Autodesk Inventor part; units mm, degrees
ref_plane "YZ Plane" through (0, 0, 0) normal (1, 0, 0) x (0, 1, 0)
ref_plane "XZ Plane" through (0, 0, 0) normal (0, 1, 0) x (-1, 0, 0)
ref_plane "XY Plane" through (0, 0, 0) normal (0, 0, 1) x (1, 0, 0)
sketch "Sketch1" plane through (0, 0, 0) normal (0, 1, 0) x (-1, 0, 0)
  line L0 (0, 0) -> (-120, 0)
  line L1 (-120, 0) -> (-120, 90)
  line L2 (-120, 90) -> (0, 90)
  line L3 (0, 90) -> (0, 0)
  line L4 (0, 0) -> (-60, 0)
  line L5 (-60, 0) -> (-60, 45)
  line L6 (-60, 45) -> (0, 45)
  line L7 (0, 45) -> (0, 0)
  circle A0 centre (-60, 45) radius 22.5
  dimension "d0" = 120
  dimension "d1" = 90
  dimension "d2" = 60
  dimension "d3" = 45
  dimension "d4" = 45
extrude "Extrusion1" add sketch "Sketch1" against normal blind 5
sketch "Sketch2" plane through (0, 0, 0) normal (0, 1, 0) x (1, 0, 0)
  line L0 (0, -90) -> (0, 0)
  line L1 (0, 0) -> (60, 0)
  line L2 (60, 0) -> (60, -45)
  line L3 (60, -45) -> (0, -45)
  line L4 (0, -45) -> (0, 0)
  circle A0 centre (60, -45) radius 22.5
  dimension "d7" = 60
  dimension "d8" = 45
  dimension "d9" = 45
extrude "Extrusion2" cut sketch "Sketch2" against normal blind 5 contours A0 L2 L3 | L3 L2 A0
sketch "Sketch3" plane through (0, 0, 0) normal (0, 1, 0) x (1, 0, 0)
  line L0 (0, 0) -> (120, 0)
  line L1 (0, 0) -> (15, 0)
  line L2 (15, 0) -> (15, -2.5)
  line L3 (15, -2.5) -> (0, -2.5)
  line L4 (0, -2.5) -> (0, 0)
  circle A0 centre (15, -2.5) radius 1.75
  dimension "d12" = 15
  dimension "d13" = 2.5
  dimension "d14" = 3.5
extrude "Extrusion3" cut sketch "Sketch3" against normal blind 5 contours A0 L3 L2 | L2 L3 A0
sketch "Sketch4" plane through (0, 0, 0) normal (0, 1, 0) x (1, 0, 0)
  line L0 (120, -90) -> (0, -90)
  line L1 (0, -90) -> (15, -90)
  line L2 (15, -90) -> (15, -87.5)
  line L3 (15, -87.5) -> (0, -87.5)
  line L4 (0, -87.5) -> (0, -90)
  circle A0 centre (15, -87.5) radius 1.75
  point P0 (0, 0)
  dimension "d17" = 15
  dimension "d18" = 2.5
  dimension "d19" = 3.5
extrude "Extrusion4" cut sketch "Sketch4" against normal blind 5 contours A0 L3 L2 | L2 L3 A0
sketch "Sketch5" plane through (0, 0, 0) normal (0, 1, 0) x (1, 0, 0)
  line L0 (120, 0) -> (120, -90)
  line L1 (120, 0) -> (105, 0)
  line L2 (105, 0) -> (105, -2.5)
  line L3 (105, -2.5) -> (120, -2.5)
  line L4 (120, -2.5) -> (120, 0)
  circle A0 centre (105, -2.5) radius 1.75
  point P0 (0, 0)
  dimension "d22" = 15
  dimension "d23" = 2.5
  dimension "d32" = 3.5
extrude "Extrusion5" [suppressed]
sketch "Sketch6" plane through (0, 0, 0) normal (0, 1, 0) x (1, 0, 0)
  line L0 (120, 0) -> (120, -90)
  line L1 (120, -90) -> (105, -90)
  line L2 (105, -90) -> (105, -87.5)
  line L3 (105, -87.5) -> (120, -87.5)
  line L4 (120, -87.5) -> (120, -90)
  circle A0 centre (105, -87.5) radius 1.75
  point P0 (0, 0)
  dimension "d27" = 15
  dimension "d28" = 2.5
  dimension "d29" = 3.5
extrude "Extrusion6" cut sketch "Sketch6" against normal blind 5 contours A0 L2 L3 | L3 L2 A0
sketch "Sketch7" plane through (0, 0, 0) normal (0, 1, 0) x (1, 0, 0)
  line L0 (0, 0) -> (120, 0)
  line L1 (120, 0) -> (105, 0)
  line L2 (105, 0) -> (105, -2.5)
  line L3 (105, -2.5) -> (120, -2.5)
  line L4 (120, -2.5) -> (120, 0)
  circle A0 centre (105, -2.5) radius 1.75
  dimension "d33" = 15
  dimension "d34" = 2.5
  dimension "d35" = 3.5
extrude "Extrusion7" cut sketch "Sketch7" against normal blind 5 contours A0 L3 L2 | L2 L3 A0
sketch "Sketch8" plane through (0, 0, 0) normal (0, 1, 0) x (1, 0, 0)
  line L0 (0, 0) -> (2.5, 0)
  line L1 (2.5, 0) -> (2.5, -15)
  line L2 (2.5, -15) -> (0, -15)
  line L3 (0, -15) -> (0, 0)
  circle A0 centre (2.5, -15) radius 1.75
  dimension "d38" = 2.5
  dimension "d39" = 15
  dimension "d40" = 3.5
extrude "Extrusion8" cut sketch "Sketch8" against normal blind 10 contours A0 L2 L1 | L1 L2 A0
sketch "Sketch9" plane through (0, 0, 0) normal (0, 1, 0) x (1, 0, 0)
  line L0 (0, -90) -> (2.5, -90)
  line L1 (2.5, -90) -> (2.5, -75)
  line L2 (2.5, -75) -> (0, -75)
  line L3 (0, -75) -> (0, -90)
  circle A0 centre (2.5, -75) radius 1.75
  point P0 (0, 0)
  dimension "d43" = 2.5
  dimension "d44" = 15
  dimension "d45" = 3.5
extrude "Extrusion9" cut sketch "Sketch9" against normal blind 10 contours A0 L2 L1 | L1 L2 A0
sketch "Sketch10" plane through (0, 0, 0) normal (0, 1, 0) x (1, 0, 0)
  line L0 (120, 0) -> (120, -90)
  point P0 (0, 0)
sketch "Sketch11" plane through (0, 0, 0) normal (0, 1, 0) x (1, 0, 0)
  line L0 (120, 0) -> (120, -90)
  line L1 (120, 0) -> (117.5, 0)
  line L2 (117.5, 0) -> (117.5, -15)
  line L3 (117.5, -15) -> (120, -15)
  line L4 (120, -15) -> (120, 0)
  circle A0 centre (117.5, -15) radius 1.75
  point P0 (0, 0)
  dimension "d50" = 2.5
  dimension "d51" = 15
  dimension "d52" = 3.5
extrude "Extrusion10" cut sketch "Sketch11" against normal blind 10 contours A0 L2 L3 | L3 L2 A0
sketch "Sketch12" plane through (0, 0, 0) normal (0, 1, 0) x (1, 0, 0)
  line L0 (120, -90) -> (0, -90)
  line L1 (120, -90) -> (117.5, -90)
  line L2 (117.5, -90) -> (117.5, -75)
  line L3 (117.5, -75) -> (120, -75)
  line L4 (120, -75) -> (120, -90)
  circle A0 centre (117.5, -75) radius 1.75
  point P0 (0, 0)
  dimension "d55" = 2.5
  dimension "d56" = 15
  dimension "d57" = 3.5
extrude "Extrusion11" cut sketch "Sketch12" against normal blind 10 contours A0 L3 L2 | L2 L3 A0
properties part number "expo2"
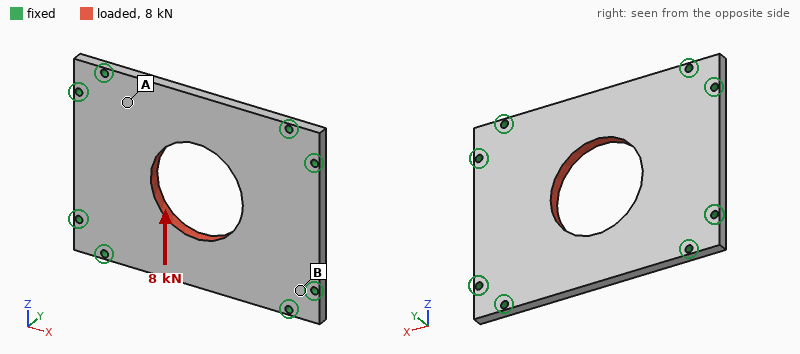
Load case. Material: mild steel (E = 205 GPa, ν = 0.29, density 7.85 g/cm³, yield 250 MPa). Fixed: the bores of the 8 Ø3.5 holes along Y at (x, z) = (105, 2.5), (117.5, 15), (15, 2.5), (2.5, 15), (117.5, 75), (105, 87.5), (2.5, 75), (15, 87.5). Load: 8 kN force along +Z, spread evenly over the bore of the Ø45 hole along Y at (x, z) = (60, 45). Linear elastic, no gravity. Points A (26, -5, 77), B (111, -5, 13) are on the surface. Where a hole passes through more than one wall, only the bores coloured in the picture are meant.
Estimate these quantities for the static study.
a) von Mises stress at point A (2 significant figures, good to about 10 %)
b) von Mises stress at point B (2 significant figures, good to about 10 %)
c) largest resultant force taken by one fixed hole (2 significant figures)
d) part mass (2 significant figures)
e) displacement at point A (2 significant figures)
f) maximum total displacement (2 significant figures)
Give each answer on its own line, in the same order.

17 MPa
7.3 MPa
1.6 kN
360 g
2.3 µm
7.1 µm
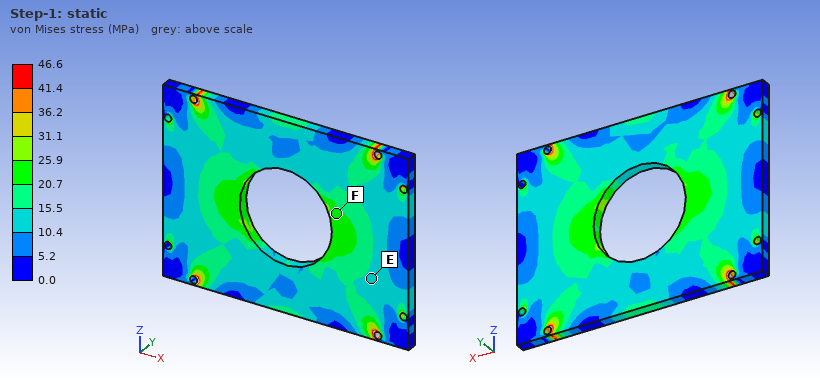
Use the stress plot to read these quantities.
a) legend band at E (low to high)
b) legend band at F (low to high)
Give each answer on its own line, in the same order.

10.4 to 15.5 MPa
20.7 to 25.9 MPa
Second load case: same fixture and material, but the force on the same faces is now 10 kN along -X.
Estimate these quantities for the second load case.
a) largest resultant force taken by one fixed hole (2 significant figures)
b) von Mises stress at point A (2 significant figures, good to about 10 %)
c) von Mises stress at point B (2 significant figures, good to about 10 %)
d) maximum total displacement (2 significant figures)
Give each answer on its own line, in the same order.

1.5 kN
15 MPa
18 MPa
4.5 µm
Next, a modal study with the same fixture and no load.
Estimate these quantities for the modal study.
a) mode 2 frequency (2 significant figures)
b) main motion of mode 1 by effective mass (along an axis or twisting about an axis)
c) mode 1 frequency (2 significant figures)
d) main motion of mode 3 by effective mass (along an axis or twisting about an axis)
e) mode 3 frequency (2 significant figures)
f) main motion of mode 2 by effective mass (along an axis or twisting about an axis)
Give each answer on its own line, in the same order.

3400 Hz
along Y
2400 Hz
twisting about Z
4500 Hz
twisting about X
